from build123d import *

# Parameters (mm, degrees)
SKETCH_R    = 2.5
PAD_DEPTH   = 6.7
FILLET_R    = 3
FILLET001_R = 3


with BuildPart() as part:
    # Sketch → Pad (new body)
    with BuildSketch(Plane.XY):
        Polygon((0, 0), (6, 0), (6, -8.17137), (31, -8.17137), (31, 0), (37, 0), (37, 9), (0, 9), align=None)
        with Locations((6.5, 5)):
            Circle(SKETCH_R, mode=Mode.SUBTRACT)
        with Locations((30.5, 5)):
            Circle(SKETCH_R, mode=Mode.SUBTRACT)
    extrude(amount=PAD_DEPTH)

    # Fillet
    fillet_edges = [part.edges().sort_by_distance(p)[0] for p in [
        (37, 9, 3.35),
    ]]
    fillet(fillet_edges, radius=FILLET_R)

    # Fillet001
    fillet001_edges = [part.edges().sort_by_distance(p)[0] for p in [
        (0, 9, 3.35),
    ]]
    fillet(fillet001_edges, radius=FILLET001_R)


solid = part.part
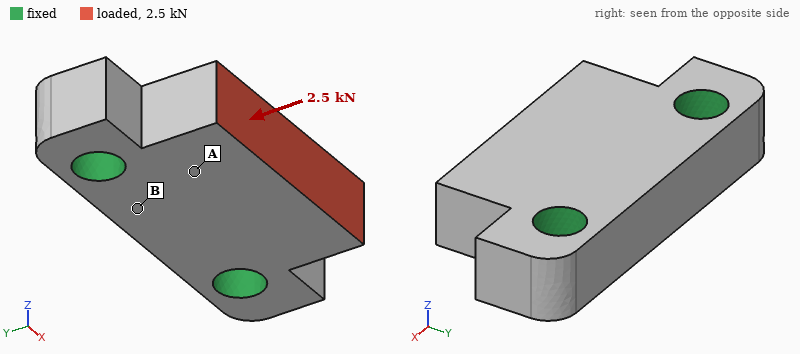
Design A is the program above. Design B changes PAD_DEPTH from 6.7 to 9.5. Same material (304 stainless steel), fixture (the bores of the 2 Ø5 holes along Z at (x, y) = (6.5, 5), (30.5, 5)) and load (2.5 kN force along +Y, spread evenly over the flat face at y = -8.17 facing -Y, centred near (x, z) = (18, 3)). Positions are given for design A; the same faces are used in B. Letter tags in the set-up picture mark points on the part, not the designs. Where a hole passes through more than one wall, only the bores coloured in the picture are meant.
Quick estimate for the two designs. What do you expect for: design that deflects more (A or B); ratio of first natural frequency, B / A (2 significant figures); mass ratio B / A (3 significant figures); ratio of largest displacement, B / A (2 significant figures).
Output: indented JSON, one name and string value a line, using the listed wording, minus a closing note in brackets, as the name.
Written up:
{
  "design that deflects more": "A",
  "ratio of first natural frequency, B / A": "1.2",
  "mass ratio B / A": "1.42",
  "ratio of largest displacement, B / A": "0.71"
}
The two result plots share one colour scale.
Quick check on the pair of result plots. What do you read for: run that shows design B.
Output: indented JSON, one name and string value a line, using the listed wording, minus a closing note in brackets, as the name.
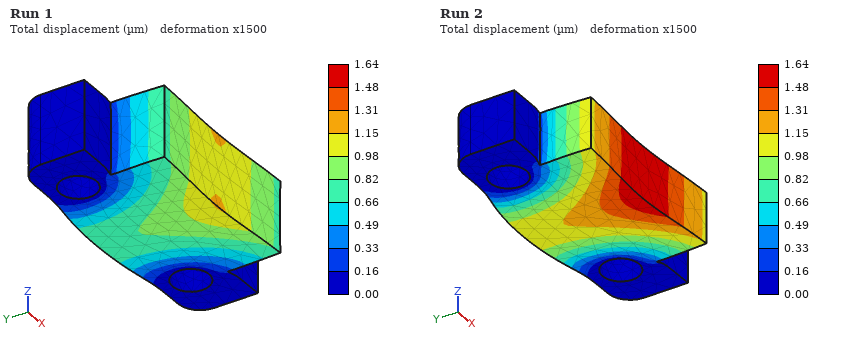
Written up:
{
  "run that shows design B": "Run 1"
}
